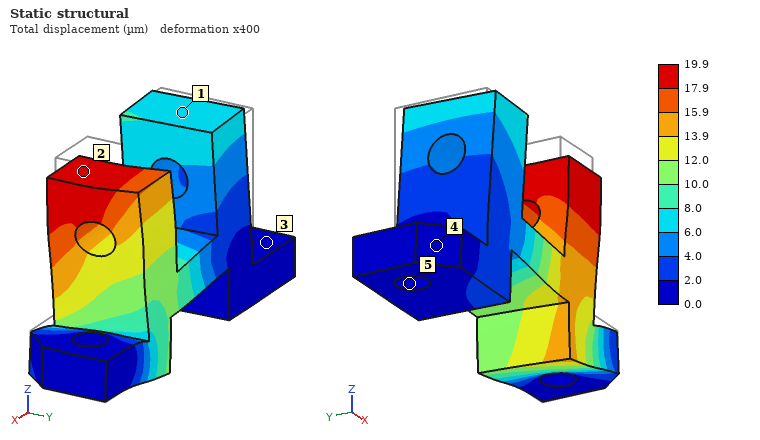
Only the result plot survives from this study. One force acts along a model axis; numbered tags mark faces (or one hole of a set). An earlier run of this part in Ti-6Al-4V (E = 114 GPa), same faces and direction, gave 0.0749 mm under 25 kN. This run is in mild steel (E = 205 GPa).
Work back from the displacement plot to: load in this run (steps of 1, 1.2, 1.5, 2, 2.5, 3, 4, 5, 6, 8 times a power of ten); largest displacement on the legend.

12 kN
19.9 µm
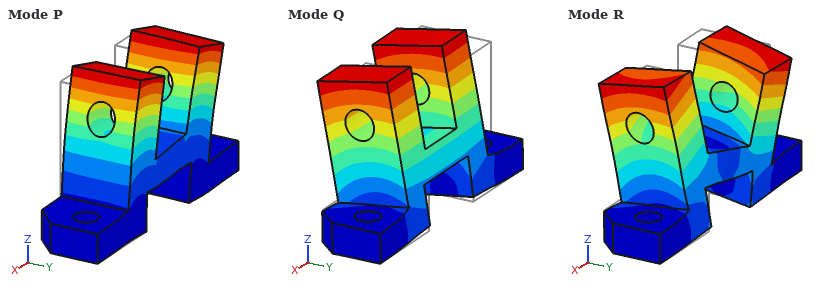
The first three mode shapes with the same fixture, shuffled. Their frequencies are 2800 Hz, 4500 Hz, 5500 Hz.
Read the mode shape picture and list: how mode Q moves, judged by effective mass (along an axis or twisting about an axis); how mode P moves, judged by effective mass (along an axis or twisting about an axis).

along Y
along X
